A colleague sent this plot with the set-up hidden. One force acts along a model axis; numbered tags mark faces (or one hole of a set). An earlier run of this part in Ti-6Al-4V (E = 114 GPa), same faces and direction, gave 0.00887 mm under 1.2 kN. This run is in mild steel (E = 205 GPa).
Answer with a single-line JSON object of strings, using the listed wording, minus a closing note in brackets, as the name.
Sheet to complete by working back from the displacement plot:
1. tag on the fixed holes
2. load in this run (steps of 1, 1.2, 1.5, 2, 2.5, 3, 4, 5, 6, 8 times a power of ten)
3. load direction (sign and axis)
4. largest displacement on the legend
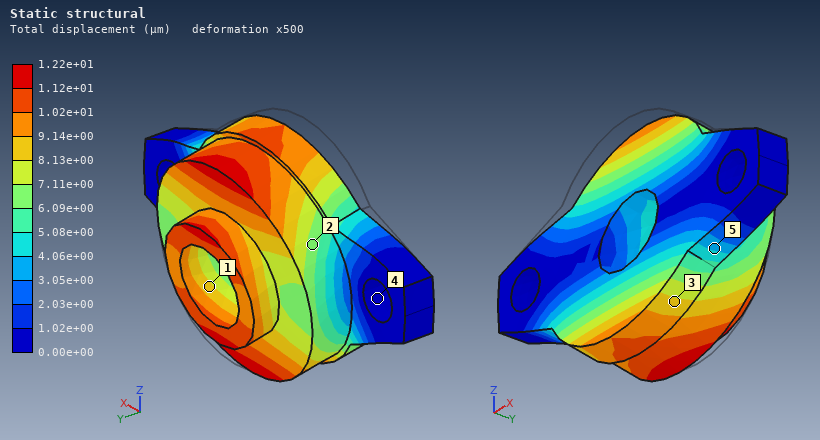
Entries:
{"tag on the fixed holes": "4", "load in this run": "3 kN", "load direction": "-Z", "largest displacement on the legend": "1.22e+01 µm"}
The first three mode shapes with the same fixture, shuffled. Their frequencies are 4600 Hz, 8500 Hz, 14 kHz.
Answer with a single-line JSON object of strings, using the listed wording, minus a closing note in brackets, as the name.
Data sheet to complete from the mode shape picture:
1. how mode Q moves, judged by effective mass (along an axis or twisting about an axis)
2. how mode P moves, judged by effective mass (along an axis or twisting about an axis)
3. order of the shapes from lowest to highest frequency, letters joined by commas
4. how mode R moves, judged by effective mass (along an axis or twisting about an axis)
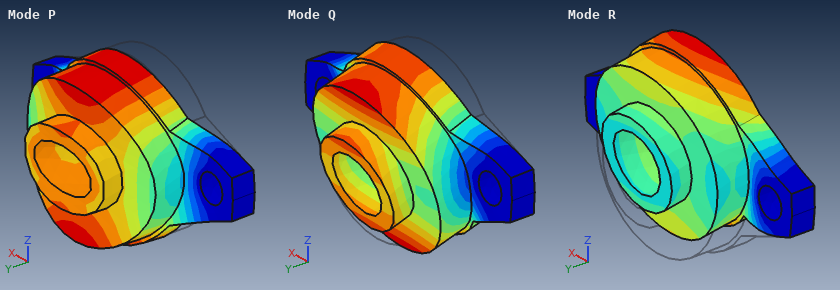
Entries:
{"how mode Q moves, judged by effective mass": "along Z", "how mode P moves, judged by effective mass": "along Y", "order of the shapes from lowest to highest frequency, letters joined by commas": "Q, P, R", "how mode R moves, judged by effective mass": "along Z"}
